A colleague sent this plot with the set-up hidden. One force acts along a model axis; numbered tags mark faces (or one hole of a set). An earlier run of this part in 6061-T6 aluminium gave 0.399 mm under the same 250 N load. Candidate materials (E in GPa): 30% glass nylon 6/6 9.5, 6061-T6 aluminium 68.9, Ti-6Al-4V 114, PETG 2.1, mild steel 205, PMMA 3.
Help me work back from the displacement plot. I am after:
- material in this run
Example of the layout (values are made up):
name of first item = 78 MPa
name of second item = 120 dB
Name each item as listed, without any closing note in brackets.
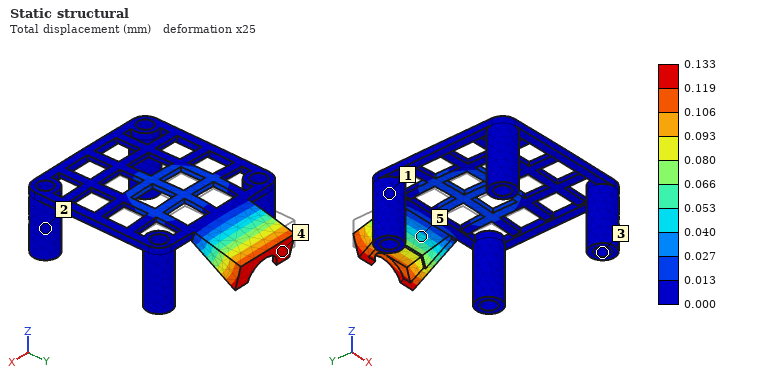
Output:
material in this run = mild steel
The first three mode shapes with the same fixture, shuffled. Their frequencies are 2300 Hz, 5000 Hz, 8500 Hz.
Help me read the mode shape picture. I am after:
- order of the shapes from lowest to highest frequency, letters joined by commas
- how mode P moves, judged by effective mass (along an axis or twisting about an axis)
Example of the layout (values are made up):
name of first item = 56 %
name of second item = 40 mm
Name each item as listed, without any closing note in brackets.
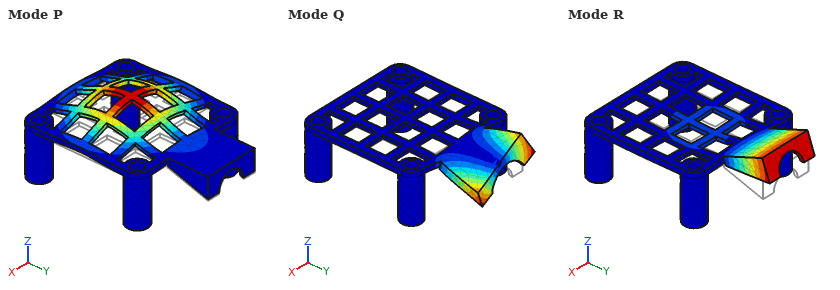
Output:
order of the shapes from lowest to highest frequency, letters joined by commas = R, P, Q
how mode P moves, judged by effective mass = along Z
